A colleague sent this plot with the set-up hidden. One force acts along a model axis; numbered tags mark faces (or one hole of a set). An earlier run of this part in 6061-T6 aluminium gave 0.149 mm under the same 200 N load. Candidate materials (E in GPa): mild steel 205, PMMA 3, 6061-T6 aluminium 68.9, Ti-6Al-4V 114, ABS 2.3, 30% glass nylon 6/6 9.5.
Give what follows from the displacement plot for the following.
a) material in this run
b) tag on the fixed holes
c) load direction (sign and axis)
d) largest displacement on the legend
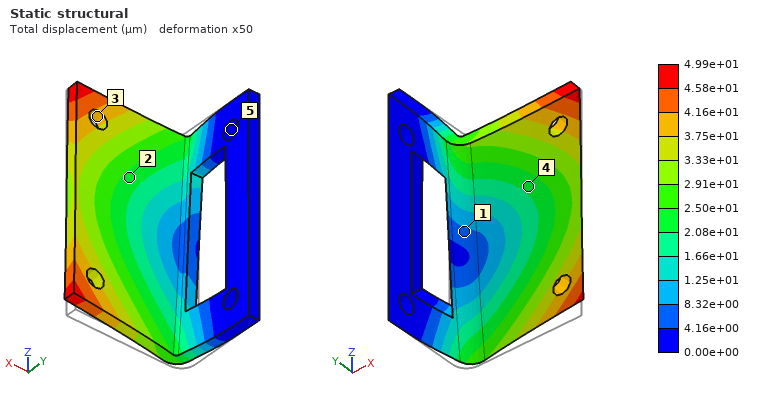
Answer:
mild steel
5
+Z
4.99e+01 µm
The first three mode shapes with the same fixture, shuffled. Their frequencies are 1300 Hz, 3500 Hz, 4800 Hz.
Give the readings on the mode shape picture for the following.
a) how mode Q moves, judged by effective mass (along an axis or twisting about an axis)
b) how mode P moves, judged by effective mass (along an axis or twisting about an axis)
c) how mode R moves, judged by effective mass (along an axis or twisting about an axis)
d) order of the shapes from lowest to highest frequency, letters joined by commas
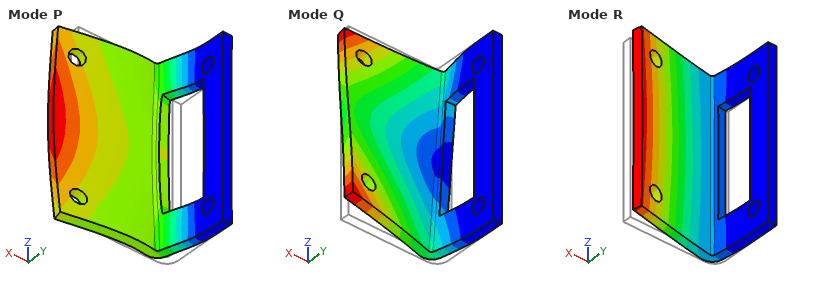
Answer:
along Z
along X
along Y
R, Q, P
